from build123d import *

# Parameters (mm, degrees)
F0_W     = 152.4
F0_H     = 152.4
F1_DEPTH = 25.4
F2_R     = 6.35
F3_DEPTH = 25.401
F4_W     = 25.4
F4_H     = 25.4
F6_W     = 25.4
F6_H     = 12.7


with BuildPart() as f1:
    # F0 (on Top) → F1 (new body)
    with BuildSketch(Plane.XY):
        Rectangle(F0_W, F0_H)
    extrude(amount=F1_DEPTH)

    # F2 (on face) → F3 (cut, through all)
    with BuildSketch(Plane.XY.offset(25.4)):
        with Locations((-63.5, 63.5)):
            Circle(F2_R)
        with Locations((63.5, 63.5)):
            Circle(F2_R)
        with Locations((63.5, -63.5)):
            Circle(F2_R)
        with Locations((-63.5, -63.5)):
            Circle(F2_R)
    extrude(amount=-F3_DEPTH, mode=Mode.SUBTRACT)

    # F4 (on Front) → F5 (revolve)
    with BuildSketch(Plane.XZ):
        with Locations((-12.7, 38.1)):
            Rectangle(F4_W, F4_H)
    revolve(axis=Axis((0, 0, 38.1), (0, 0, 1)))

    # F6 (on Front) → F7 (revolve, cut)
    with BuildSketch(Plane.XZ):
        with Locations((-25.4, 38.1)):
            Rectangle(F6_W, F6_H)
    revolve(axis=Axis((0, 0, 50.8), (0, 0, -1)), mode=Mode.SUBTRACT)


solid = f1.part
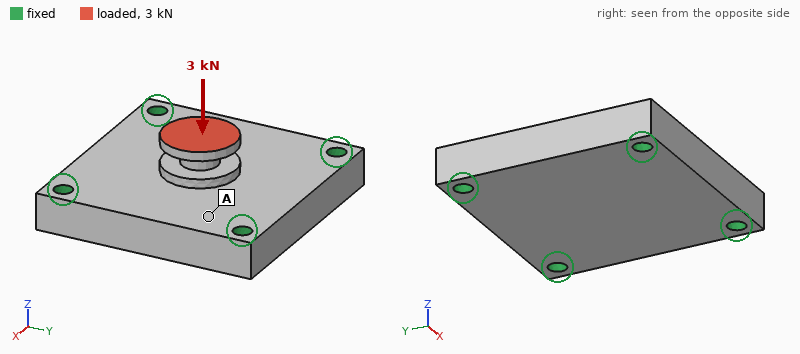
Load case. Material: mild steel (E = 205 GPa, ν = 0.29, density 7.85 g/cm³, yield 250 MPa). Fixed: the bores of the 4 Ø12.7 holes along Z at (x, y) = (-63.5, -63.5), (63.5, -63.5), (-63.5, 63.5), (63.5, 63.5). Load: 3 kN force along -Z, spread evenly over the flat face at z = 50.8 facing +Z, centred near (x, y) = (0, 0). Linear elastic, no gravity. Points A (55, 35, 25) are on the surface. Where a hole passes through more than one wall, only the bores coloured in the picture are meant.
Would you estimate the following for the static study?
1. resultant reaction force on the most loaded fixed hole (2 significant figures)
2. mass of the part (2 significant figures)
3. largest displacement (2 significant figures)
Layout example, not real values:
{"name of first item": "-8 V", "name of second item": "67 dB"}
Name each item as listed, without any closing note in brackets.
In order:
{"resultant reaction force on the most loaded fixed hole": "760 N", "mass of the part": "4.8 kg", "largest displacement": "5.5 µm"}
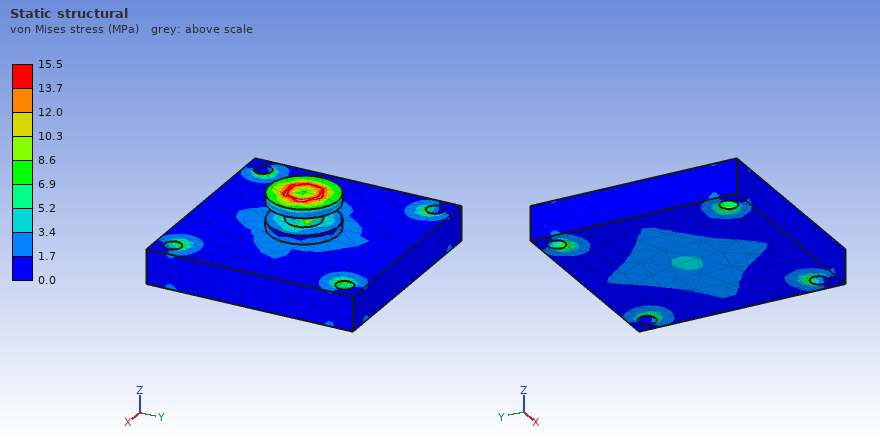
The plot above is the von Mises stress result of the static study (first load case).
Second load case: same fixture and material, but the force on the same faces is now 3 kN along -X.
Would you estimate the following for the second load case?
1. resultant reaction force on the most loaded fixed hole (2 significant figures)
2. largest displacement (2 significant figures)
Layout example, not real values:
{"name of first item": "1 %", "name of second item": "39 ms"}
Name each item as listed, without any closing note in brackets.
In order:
{"resultant reaction force on the most loaded fixed hole": "1000 N", "largest displacement": "11 µm"}
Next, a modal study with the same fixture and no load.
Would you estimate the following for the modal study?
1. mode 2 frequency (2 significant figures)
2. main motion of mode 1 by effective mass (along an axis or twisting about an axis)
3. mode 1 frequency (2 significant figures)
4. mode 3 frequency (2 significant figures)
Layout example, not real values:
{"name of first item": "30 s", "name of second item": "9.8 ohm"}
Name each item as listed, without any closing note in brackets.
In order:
{"mode 2 frequency": "7000 Hz", "main motion of mode 1 by effective mass": "along Z", "mode 1 frequency": "4400 Hz", "mode 3 frequency": "7000 Hz"}
